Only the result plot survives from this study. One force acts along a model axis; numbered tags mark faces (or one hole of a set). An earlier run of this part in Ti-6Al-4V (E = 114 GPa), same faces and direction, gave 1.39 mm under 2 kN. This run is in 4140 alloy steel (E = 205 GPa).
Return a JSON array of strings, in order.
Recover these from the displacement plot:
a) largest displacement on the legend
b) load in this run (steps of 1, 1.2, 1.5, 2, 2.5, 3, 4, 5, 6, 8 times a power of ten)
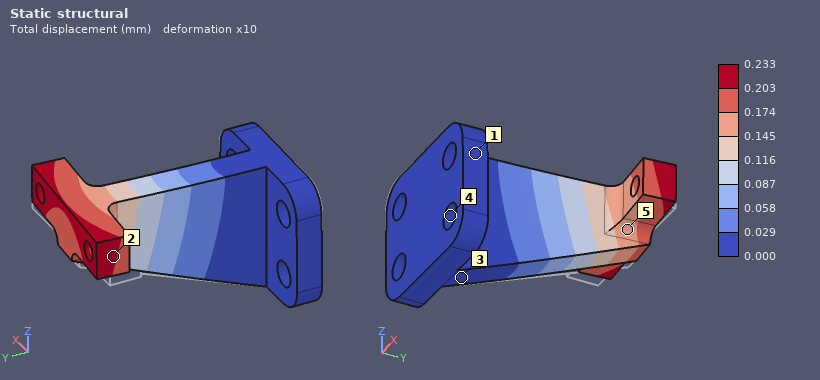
["0.233 mm", "600 N"]
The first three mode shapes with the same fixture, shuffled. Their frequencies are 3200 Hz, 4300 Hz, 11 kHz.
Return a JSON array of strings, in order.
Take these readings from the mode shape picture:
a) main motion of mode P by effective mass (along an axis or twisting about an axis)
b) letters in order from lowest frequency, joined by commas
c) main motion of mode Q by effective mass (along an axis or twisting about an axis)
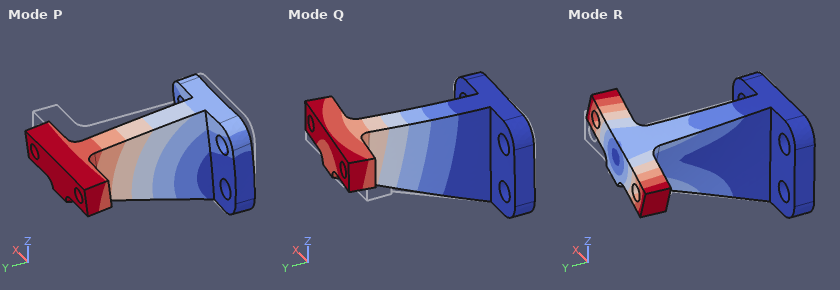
["along Z", "Q, P, R", "along X"]
